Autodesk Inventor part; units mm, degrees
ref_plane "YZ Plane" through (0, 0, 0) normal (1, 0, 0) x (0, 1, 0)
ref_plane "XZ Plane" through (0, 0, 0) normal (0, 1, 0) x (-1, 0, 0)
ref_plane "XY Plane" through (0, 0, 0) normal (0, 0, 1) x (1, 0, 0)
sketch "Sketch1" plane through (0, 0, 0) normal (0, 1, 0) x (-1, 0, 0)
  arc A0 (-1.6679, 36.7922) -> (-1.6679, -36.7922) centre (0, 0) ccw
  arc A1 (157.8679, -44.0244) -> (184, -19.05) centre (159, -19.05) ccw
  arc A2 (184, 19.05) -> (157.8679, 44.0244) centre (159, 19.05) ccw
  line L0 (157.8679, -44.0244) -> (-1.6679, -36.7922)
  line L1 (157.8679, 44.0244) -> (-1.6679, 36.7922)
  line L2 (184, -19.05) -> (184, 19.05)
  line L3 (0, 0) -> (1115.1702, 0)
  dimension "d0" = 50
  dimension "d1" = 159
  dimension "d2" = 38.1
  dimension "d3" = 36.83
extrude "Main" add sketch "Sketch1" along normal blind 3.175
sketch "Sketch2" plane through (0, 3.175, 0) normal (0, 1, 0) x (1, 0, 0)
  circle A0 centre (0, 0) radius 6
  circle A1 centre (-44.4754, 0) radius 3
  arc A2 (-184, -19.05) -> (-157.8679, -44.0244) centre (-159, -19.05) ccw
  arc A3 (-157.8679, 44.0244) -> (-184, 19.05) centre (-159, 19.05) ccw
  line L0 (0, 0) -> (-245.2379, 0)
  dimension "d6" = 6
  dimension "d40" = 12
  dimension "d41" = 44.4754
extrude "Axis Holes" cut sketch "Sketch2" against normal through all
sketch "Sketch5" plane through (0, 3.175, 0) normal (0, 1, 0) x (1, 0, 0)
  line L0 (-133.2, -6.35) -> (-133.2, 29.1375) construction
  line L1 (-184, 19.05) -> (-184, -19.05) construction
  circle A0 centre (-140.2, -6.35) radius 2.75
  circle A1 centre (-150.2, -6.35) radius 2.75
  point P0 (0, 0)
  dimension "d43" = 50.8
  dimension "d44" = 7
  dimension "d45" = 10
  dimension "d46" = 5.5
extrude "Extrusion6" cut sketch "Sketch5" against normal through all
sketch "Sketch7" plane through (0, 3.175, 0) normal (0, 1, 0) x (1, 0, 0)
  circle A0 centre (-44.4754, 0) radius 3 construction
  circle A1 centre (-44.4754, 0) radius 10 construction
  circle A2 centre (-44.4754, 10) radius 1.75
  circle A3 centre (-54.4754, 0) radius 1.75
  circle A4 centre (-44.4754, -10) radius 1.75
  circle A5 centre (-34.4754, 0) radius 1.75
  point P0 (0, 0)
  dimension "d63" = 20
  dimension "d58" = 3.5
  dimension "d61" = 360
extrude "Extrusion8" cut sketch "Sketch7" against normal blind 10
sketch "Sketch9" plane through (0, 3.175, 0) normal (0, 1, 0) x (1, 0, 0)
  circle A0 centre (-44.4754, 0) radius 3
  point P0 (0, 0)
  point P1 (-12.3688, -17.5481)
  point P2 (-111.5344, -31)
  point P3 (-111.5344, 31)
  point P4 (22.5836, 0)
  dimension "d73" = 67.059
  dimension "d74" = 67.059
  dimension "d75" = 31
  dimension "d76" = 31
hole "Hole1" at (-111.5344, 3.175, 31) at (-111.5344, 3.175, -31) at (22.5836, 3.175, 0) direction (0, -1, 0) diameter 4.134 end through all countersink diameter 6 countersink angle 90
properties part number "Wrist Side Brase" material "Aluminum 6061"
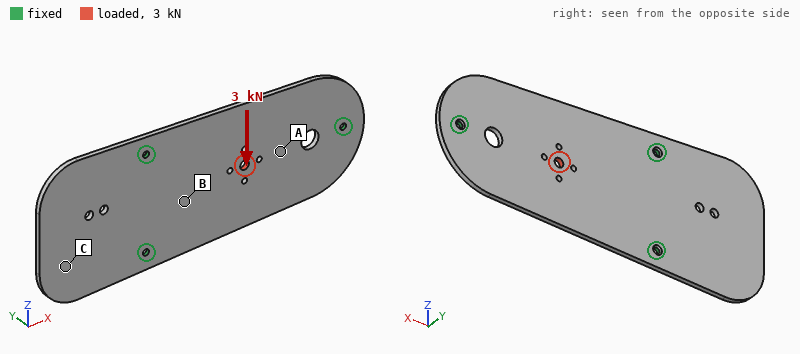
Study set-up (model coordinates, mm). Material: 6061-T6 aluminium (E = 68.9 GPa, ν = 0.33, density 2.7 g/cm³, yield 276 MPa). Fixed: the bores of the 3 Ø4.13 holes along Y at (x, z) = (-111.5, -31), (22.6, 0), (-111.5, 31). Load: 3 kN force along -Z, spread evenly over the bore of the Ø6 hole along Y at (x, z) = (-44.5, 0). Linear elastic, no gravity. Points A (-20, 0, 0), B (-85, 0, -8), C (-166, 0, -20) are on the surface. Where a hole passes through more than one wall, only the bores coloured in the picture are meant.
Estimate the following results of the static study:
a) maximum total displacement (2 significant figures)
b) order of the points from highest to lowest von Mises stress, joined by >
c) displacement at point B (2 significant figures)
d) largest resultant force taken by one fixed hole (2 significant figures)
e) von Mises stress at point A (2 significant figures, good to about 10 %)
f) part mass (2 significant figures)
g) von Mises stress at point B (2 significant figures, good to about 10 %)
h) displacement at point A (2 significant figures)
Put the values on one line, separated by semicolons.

36 µm; B > A > C; 13 µm; 1.4 kN; 9.9 MPa; 140 g; 18 MPa; 24 µm
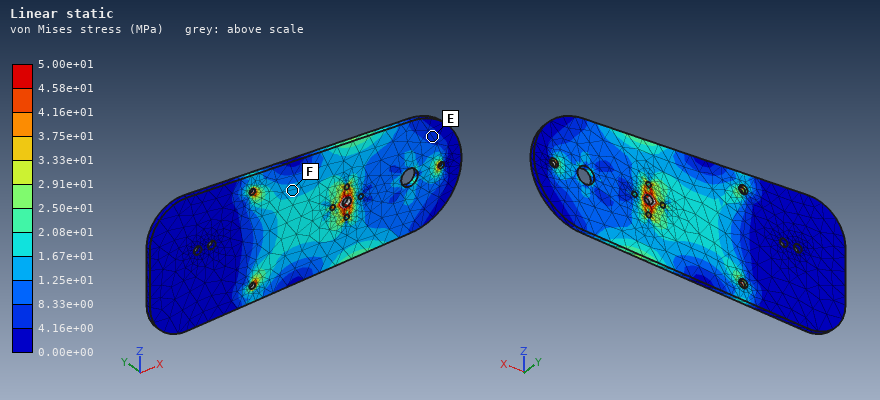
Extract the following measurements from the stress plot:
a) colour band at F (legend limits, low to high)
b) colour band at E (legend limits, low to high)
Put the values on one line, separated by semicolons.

1.25e+01 to 1.67e+01 MPa; 4.16e+00 to 8.33e+00 MPa
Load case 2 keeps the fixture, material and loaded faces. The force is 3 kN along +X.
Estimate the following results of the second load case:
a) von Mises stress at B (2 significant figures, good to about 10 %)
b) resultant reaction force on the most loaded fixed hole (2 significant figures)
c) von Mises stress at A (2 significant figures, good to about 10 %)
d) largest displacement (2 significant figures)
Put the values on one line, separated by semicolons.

8.8 MPa; 1.1 kN; 11 MPa; 18 µm
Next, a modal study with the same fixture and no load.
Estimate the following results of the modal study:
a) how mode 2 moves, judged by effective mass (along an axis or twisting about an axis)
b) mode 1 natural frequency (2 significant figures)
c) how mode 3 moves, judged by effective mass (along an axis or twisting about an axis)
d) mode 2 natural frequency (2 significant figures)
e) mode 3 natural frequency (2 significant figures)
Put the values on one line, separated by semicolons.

along Y; 460 Hz; twisting about X; 760 Hz; 990 Hz
